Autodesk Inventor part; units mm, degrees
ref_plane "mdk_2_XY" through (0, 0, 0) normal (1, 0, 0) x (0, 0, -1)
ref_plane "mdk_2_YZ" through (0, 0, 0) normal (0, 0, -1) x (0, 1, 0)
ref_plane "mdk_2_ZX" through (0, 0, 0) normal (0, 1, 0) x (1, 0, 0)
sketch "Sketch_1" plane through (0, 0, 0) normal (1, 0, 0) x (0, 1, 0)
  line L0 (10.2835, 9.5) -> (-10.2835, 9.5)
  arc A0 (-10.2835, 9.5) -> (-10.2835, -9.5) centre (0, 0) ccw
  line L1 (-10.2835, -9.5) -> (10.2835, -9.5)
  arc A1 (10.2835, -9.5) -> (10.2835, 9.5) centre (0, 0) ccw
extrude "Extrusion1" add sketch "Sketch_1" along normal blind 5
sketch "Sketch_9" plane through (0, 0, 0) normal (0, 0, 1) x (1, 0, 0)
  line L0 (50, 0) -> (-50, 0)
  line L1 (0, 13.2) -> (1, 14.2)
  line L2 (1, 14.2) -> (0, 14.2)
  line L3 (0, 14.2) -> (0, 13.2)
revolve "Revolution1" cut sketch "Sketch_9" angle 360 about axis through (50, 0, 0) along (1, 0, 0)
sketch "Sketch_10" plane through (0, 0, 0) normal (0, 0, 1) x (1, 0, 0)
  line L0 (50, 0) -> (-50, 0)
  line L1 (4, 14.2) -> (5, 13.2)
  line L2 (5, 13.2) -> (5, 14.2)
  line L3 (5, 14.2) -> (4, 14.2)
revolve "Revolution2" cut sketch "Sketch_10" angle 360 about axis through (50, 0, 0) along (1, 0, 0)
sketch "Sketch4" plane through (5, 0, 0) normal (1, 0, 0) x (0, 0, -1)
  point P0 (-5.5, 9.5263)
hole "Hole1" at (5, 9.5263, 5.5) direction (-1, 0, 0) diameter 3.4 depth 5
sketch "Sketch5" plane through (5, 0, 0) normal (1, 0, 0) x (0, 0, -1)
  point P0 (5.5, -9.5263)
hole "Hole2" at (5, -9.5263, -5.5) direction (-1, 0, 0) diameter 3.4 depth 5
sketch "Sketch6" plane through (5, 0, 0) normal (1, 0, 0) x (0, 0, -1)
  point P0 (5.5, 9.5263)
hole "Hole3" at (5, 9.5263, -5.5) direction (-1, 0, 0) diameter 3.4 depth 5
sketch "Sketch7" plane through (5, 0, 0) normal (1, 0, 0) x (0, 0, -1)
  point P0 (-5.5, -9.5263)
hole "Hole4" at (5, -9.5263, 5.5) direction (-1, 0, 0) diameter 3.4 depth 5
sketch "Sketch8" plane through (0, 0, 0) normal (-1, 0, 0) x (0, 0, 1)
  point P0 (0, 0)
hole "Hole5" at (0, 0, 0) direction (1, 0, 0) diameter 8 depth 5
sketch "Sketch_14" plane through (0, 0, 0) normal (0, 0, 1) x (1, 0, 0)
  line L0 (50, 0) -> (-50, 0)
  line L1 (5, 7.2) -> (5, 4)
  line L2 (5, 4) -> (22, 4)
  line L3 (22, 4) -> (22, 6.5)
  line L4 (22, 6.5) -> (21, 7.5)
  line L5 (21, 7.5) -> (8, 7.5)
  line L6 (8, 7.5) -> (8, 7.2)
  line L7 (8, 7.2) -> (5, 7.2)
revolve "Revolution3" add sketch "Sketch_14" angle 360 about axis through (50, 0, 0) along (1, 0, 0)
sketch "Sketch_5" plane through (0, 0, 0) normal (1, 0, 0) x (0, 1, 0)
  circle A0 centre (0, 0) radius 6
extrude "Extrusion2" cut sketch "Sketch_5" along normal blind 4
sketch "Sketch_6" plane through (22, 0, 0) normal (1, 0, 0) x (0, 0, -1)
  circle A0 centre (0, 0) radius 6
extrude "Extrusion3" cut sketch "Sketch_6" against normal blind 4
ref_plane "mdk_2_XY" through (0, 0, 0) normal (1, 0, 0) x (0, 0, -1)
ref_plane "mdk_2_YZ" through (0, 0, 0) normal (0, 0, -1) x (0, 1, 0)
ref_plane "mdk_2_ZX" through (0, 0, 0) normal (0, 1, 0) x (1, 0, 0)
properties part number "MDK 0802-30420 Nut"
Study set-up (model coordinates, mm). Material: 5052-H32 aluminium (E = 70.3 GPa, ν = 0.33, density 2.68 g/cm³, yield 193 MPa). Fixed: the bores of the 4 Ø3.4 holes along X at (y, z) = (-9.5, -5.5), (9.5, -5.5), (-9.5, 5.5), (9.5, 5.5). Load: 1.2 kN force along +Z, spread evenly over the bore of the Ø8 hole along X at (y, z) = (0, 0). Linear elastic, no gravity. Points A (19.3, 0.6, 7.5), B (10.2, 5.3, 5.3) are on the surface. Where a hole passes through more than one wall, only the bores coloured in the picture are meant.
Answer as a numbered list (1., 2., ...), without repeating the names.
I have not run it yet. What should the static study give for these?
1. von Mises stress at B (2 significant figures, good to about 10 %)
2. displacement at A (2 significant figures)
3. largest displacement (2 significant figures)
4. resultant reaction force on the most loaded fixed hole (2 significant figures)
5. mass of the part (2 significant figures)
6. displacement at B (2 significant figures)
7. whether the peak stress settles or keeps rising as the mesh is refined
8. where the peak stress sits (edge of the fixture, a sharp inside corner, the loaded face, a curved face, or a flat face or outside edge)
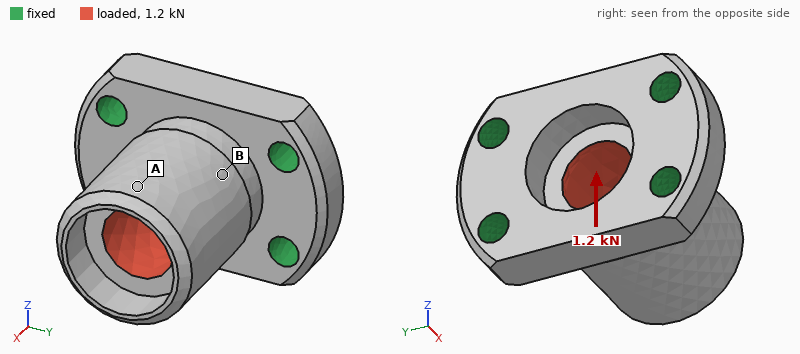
1. 9.7 MPa
2. 18 µm
3. 20 µm
4. 530 N
5. 9.5 g
6. 9.3 µm
7. keeps rising
8. edge of the fixture
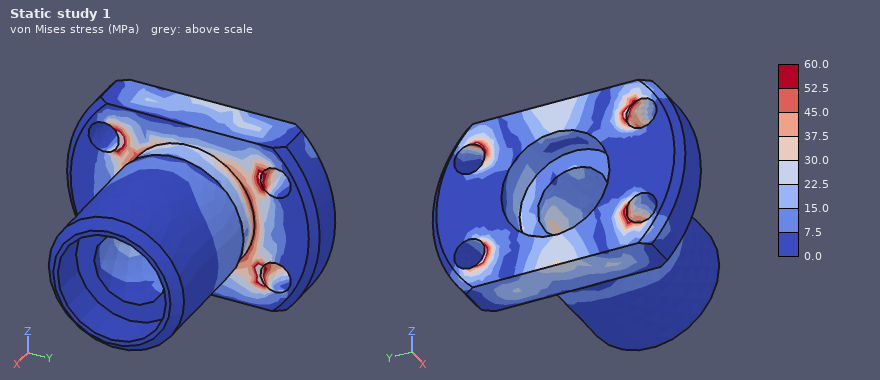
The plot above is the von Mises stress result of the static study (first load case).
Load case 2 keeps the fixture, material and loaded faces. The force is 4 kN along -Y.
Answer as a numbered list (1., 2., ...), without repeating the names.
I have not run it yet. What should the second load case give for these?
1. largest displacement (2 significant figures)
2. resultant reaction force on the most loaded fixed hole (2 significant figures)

1. 41 µm
2. 1.5 kN
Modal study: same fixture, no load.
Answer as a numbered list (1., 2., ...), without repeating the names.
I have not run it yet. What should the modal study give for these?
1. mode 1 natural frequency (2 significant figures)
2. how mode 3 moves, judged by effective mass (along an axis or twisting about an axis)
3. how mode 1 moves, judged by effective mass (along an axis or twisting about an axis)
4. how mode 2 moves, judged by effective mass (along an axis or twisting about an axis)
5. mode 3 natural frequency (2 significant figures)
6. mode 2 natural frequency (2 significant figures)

1. 18 kHz
2. twisting about X
3. along Z
4. along Y
5. 42 kHz
6. 23 kHz
